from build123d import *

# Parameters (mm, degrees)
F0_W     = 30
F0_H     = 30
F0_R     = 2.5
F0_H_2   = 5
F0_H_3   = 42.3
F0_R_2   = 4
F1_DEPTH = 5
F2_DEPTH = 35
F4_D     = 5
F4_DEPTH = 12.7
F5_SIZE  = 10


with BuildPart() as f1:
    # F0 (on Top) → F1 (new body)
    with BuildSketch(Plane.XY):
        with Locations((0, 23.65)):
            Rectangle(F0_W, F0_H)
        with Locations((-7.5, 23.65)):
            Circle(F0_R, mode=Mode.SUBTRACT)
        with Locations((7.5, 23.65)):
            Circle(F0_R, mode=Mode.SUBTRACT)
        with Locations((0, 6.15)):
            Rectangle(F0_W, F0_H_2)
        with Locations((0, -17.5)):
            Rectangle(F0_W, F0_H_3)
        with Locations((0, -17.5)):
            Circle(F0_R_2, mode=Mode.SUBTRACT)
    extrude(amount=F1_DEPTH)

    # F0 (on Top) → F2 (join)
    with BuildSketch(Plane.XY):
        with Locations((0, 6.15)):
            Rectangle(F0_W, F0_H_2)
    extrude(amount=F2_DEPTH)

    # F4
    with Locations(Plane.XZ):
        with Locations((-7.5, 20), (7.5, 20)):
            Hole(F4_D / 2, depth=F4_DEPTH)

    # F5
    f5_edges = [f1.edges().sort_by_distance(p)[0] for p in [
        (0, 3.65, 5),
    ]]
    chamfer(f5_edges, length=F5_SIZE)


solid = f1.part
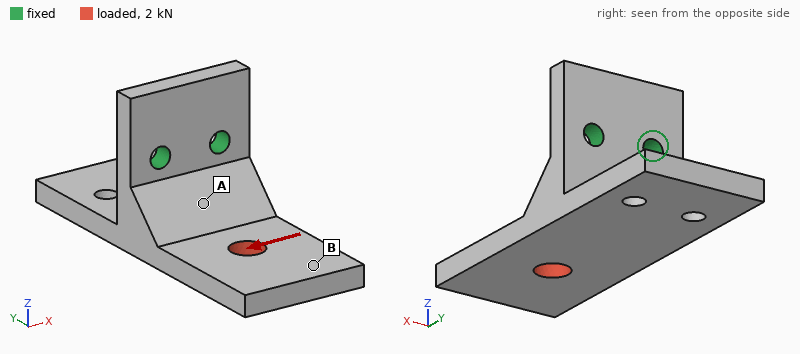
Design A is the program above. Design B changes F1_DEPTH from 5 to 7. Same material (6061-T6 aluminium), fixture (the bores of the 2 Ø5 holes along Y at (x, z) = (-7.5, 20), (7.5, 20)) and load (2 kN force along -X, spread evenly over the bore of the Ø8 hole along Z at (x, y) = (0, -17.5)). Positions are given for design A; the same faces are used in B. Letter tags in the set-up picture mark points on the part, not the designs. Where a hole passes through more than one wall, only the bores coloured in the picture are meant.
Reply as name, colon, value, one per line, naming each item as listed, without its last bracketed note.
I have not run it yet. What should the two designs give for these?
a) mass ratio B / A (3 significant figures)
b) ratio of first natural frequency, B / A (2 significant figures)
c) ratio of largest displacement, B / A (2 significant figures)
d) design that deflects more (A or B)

mass ratio B / A: 1.25
ratio of first natural frequency, B / A: 1.0
ratio of largest displacement, B / A: 0.69
design that deflects more: A
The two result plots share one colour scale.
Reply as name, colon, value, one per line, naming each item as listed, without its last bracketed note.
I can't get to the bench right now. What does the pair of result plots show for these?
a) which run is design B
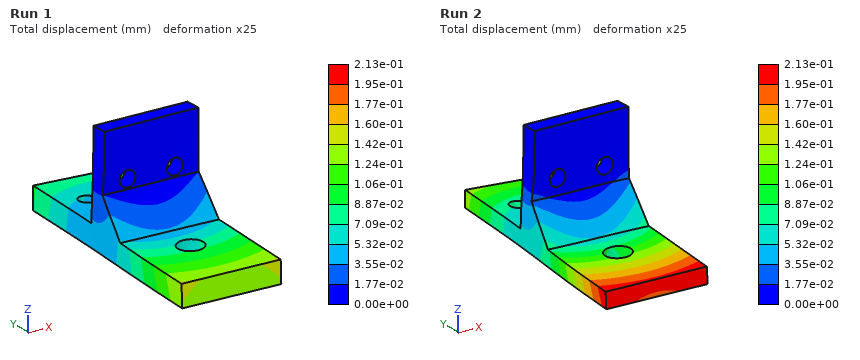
which run is design B: Run 1
